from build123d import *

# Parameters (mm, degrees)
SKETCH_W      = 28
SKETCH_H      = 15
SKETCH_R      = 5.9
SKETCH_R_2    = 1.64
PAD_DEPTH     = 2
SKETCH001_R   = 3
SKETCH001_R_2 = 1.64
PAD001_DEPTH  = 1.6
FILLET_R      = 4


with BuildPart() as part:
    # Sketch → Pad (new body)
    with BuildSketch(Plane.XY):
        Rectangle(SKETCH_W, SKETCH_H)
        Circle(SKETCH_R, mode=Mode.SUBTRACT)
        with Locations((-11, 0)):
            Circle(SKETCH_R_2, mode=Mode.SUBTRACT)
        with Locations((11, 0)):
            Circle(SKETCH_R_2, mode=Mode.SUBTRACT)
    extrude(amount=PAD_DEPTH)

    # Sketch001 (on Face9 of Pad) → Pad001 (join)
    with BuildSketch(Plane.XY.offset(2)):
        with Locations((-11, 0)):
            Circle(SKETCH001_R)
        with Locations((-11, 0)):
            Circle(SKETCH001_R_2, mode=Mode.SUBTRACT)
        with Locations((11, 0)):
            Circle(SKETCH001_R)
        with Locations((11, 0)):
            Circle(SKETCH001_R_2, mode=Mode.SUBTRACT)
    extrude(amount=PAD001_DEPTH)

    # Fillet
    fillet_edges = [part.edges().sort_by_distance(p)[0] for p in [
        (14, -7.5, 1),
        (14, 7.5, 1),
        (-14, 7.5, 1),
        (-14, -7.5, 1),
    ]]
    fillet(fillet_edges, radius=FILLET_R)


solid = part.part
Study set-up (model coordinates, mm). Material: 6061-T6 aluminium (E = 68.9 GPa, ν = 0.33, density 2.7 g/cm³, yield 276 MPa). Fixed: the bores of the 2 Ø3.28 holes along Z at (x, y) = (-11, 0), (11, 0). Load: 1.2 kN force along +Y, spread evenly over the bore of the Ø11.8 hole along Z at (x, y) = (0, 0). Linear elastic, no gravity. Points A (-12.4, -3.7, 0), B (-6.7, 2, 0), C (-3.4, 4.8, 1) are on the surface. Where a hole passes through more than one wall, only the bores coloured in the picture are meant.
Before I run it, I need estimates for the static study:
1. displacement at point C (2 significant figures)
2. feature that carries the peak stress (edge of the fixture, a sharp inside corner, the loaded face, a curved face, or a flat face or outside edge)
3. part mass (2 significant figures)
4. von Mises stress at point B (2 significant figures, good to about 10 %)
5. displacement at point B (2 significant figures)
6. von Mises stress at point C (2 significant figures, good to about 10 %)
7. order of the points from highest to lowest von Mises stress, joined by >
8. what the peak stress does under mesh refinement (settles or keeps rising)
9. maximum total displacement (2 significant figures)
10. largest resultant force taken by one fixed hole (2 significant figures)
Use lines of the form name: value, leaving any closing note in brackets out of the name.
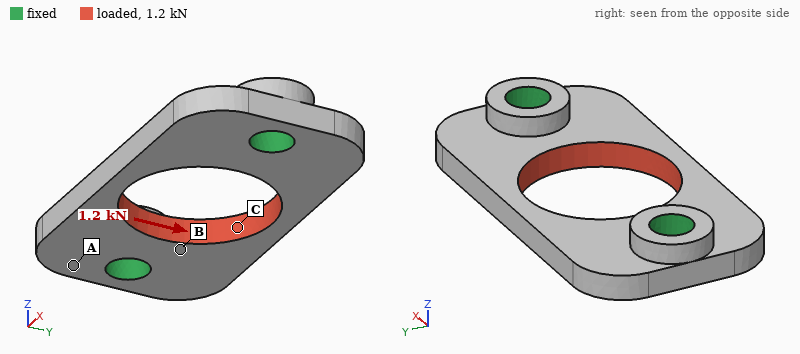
displacement at point C: 12 µm
feature that carries the peak stress: edge of the fixture
part mass: 1.7 g
von Mises stress at point B: 56 MPa
displacement at point B: 5.2 µm
von Mises stress at point C: 86 MPa
order of the points from highest to lowest von Mises stress, joined by >: C > B > A
what the peak stress does under mesh refinement: keeps rising
maximum total displacement: 18 µm
largest resultant force taken by one fixed hole: 600 N
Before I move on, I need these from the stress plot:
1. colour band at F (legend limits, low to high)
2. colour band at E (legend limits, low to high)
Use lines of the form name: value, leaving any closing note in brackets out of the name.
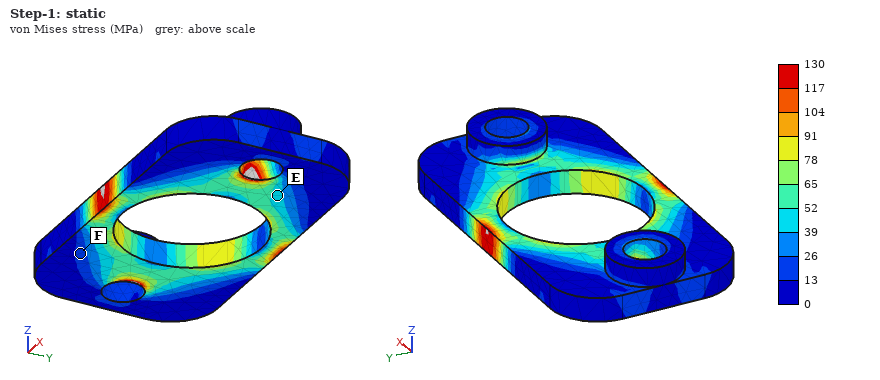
colour band at F: 13 to 26 MPa
colour band at E: 39 to 52 MPa
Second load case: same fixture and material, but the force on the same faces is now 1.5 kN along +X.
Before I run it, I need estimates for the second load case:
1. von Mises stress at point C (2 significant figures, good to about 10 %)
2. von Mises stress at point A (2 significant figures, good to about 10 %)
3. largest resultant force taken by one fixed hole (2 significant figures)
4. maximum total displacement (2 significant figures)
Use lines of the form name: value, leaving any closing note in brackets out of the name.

von Mises stress at point C: 61 MPa
von Mises stress at point A: 23 MPa
largest resultant force taken by one fixed hole: 750 N
maximum total displacement: 8.9 µm
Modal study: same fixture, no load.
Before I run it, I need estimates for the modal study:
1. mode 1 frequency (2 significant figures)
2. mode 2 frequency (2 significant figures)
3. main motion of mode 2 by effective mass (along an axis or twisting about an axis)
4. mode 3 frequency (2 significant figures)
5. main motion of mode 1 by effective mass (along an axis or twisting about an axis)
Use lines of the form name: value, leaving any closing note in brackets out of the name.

mode 1 frequency: 23 kHz
mode 2 frequency: 24 kHz
main motion of mode 2 by effective mass: along Z
mode 3 frequency: 41 kHz
main motion of mode 1 by effective mass: twisting about X
